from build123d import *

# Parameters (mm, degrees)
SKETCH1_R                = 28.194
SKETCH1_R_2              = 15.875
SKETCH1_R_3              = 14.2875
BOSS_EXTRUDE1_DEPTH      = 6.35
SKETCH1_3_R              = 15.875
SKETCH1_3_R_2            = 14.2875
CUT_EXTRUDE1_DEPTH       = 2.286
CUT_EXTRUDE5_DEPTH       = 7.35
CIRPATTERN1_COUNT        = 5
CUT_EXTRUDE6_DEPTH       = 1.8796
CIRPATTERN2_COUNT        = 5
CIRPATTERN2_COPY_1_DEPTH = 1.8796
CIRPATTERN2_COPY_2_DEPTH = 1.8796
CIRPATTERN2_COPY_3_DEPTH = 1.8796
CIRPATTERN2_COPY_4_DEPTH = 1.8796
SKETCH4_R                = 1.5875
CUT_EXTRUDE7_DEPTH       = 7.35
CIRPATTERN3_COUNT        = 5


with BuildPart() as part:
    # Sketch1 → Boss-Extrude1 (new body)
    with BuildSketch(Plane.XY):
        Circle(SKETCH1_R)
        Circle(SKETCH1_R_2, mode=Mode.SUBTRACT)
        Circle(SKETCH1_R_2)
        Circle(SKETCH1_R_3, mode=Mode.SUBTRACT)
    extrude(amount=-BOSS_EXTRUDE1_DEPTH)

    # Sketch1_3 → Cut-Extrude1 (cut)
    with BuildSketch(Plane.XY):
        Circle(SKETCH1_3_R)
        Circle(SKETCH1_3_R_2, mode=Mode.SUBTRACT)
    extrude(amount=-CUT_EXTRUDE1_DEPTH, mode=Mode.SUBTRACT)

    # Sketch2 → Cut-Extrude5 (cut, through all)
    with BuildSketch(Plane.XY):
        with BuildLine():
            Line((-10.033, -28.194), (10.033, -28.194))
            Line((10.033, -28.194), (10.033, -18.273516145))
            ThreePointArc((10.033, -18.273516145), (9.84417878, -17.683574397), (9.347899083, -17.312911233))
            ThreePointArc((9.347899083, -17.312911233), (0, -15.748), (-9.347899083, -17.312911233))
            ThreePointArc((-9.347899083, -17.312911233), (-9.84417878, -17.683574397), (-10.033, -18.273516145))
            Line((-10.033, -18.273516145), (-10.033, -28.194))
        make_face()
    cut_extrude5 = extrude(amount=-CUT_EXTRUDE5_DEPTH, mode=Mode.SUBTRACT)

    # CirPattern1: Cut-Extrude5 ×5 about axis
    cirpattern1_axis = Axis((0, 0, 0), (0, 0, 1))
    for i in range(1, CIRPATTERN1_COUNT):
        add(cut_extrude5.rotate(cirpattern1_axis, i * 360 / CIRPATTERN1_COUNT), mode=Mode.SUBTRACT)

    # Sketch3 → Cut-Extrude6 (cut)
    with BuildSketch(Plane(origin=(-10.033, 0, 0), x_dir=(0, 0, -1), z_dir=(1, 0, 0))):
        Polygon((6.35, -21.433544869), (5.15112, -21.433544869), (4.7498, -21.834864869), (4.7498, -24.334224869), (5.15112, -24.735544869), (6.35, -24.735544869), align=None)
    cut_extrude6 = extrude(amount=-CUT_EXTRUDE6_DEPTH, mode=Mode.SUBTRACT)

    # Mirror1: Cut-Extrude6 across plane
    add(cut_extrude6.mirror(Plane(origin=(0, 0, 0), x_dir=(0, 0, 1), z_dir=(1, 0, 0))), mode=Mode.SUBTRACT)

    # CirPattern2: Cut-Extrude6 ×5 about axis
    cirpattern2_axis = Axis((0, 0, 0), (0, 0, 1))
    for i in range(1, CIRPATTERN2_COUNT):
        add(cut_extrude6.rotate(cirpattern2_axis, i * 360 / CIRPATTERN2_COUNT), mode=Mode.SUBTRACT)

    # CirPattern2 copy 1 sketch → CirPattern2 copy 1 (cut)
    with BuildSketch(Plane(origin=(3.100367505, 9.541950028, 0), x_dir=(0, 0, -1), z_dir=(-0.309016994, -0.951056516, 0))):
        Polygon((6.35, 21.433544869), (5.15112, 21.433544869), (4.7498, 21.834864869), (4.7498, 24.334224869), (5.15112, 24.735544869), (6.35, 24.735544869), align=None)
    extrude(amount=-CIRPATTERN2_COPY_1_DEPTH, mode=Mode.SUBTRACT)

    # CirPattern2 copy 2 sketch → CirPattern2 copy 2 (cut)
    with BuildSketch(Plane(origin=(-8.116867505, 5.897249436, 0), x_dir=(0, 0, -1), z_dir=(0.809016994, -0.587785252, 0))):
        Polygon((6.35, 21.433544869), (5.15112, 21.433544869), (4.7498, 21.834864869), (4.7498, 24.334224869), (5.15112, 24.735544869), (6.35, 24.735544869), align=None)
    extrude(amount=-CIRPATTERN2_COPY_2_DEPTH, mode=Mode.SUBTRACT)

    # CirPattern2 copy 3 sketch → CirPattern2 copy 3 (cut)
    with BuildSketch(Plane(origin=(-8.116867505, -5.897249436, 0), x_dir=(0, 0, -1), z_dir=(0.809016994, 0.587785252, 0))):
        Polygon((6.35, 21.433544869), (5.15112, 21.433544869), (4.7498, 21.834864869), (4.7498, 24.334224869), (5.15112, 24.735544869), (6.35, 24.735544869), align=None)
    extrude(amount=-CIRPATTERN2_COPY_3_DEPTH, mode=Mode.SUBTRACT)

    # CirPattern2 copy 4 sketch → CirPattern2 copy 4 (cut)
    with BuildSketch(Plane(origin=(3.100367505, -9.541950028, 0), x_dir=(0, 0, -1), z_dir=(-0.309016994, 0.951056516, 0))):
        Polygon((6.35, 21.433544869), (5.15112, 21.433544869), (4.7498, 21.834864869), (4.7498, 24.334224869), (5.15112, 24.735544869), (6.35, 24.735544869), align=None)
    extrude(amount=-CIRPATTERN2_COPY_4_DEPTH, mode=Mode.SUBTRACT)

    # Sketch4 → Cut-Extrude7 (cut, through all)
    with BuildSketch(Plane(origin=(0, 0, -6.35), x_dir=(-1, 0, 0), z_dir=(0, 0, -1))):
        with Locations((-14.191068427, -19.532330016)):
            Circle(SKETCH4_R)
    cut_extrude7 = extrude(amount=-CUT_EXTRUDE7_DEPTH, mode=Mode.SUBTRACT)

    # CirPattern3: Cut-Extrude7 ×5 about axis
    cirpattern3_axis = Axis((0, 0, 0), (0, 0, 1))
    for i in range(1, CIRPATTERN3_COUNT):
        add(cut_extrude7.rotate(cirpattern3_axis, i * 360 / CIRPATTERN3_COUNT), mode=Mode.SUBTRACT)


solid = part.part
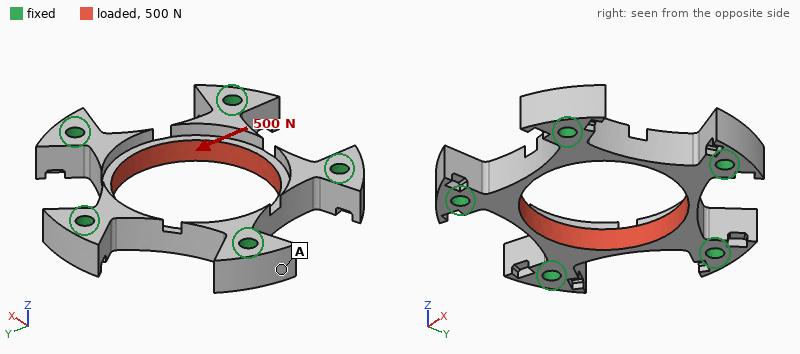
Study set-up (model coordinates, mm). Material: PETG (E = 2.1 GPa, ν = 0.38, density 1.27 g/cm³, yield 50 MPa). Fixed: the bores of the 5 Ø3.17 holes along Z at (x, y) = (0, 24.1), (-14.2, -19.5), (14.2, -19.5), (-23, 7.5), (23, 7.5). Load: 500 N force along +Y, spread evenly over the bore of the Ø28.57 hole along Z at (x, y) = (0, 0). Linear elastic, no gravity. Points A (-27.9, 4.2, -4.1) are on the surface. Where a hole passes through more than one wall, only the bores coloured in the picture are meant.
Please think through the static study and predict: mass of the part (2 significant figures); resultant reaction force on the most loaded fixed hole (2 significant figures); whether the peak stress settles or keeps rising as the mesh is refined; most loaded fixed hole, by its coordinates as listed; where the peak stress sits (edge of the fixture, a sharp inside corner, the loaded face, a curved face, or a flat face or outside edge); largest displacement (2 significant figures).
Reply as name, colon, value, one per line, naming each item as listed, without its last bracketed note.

mass of the part: 5.0 g
resultant reaction force on the most loaded fixed hole: 140 N
whether the peak stress settles or keeps rising as the mesh is refined: keeps rising
most loaded fixed hole, by its coordinates as listed: (0, 24.1)
where the peak stress sits: a sharp inside corner
largest displacement: 0.18 mm
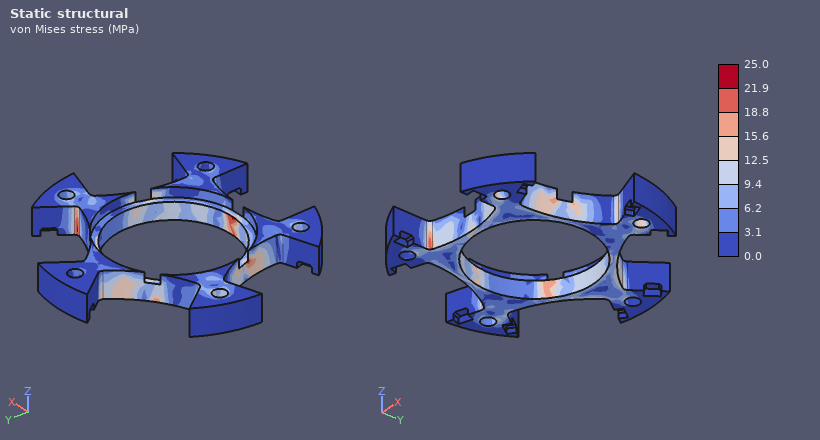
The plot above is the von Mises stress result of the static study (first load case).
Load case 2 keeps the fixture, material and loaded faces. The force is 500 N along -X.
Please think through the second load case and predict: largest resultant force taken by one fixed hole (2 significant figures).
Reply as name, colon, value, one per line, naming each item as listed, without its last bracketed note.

largest resultant force taken by one fixed hole: 140 N
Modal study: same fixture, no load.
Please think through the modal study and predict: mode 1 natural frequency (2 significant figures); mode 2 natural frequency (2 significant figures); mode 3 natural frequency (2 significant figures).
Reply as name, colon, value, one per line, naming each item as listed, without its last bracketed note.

mode 1 natural frequency: 7700 Hz
mode 2 natural frequency: 7700 Hz
mode 3 natural frequency: 8700 Hz
